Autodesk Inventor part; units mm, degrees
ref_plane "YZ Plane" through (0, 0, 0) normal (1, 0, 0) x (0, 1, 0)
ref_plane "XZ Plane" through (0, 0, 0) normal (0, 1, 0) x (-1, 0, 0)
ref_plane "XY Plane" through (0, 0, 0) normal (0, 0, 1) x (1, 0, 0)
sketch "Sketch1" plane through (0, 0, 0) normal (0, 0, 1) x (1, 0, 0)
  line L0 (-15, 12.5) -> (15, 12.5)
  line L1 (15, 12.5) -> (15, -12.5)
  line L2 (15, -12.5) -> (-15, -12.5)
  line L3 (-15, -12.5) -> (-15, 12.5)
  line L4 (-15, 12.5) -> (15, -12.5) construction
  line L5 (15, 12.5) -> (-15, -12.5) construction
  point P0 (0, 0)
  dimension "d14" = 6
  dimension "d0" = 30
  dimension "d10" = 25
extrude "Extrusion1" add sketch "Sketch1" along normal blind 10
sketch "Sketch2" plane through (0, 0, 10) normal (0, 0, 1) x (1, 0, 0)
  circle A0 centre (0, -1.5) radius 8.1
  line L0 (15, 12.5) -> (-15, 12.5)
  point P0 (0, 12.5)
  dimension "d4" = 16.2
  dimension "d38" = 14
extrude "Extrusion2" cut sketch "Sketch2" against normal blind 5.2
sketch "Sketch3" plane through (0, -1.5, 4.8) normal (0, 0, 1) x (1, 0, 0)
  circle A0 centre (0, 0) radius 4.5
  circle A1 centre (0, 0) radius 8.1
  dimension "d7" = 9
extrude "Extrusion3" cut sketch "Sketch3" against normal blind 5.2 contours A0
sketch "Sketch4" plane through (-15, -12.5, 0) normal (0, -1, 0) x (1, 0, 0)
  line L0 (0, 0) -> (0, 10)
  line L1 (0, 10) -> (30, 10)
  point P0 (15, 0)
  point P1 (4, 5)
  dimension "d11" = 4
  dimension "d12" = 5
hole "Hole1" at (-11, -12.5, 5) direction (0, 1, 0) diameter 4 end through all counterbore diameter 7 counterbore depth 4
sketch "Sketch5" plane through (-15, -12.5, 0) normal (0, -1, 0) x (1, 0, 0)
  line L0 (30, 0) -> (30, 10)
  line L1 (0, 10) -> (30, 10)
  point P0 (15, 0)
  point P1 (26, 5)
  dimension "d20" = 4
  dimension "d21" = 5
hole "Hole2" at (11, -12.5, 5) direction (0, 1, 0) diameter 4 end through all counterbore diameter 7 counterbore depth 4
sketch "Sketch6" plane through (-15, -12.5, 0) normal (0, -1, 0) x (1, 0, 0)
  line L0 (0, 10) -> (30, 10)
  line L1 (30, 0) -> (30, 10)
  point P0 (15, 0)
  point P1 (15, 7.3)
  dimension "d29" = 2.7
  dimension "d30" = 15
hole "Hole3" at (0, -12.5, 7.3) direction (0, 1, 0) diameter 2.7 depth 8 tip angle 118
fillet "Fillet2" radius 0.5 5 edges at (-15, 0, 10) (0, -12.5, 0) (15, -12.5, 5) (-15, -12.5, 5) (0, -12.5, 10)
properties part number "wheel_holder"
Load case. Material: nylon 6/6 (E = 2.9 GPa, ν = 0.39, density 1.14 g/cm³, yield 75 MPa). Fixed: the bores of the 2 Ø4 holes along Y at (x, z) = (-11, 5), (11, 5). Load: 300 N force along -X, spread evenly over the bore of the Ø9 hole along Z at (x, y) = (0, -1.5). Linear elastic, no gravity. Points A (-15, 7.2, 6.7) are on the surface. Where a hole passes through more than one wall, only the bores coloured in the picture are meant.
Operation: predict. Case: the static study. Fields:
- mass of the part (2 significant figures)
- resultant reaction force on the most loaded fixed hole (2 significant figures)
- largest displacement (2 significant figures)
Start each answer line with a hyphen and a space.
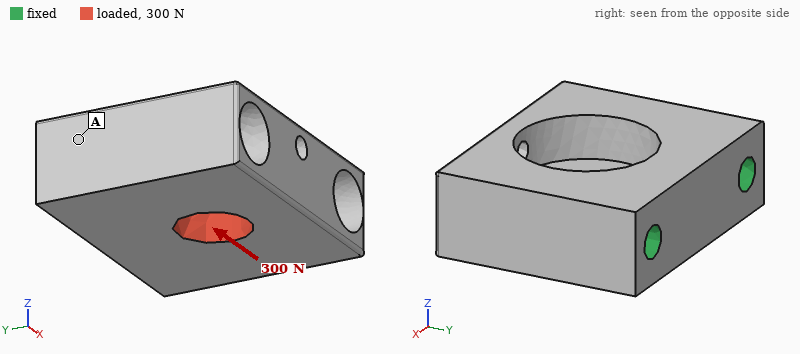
- 6.0 g
- 150 N
- 7.7 µm
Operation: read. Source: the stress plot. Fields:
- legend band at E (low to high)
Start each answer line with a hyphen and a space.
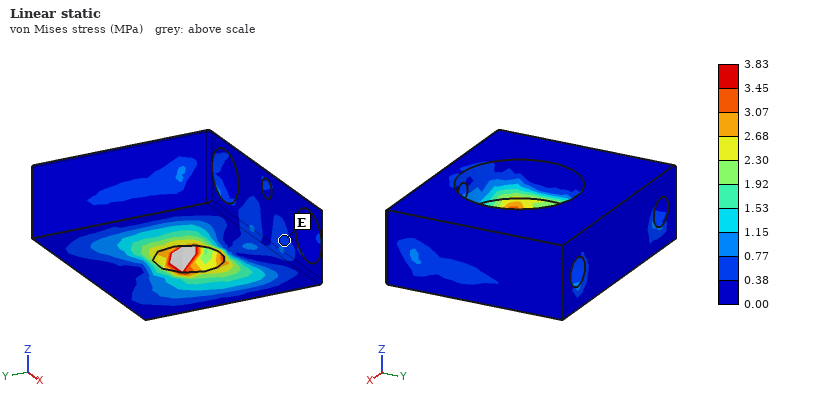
- 0.38 to 0.77 MPa
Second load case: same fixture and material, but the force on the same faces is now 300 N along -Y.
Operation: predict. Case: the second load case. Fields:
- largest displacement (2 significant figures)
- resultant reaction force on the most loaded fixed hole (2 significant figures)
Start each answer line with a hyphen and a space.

- 17 µm
- 150 N
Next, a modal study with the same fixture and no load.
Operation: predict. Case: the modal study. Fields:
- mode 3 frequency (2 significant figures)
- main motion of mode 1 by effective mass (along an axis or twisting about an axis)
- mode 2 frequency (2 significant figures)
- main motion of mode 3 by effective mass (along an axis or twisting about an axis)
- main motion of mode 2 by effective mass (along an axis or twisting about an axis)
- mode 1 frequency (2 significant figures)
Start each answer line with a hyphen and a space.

- 21 kHz
- along Z
- 19 kHz
- along Y
- along Z
- 14 kHz
